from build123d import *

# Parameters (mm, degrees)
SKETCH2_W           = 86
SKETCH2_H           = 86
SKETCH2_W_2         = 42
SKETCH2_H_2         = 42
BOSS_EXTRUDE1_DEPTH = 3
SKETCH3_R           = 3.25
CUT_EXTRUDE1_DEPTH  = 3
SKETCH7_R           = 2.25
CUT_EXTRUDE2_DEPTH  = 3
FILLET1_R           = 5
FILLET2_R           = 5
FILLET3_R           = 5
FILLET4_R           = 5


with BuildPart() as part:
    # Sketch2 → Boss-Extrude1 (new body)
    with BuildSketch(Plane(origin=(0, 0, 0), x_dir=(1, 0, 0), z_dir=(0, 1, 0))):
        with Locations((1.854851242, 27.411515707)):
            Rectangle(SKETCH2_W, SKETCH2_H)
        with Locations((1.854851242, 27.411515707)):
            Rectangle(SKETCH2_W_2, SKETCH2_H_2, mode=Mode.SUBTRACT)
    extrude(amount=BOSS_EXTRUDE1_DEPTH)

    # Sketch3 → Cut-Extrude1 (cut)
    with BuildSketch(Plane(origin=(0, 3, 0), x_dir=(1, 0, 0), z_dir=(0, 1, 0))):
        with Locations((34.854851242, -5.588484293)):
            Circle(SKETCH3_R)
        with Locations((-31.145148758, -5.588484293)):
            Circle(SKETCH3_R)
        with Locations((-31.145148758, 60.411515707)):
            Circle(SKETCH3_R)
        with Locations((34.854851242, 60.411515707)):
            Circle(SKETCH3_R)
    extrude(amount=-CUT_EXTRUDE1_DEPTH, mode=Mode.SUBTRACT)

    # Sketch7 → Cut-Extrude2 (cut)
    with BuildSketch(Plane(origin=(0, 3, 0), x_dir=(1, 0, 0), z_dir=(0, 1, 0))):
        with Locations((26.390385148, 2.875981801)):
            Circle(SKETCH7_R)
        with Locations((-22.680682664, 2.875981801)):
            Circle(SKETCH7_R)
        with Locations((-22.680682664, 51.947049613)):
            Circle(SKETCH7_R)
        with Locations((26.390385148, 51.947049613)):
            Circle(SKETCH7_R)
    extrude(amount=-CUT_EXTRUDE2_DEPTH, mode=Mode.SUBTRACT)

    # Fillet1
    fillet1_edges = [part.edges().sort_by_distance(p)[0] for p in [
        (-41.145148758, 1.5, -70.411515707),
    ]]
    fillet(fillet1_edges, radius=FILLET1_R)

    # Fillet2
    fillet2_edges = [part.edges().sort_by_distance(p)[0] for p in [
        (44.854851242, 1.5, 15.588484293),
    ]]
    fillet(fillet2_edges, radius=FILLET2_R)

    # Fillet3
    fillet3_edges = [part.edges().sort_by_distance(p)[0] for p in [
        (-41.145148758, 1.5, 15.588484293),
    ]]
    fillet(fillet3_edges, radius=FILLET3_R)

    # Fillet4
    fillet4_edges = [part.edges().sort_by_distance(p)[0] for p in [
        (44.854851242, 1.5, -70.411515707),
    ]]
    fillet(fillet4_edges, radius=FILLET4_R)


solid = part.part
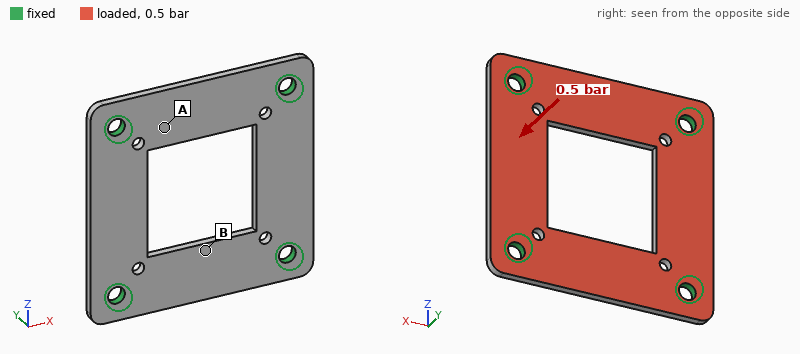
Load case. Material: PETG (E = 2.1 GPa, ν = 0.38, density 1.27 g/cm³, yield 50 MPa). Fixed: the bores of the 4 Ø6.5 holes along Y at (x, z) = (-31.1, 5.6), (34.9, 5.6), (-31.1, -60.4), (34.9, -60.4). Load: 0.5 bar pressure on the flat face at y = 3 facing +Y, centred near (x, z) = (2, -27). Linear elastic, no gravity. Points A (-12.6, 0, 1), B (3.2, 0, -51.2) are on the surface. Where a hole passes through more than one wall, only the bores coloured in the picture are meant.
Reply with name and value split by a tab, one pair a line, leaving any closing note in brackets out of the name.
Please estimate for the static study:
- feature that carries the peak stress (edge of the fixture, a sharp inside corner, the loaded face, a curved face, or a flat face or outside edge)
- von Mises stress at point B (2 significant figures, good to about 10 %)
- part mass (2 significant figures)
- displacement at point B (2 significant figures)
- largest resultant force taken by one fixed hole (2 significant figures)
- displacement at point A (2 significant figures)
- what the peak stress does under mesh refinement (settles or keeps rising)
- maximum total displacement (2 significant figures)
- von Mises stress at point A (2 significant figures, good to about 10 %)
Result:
feature that carries the peak stress	edge of the fixture
von Mises stress at point B	5.0 MPa
part mass	21 g
displacement at point B	0.50 mm
largest resultant force taken by one fixed hole	68 N
displacement at point A	0.30 mm
what the peak stress does under mesh refinement	keeps rising
maximum total displacement	0.53 mm
von Mises stress at point A	2.5 MPa
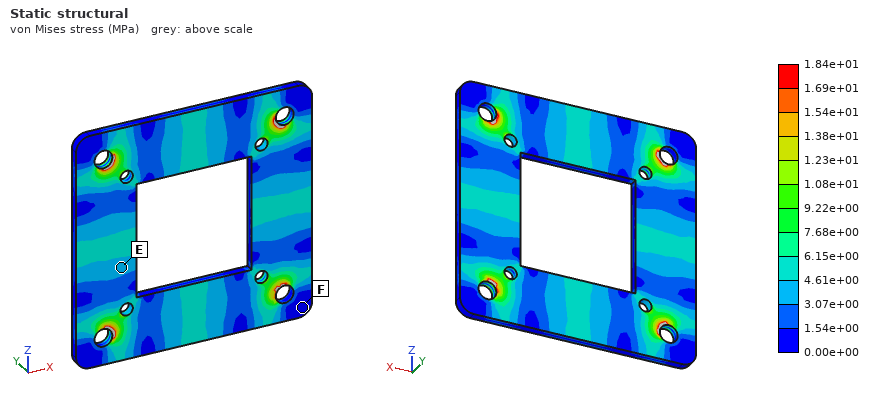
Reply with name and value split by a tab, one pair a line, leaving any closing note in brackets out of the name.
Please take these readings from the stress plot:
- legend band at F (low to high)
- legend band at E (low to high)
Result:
legend band at F	0.00e+00 to 1.54e+00 MPa
legend band at E	3.07e+00 to 4.61e+00 MPa
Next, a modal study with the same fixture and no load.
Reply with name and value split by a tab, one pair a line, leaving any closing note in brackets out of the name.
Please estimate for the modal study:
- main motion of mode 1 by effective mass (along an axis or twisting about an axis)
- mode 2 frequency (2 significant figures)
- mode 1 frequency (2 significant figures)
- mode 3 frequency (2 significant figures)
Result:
main motion of mode 1 by effective mass	along Y
mode 2 frequency	1000 Hz
mode 1 frequency	980 Hz
mode 3 frequency	1000 Hz
